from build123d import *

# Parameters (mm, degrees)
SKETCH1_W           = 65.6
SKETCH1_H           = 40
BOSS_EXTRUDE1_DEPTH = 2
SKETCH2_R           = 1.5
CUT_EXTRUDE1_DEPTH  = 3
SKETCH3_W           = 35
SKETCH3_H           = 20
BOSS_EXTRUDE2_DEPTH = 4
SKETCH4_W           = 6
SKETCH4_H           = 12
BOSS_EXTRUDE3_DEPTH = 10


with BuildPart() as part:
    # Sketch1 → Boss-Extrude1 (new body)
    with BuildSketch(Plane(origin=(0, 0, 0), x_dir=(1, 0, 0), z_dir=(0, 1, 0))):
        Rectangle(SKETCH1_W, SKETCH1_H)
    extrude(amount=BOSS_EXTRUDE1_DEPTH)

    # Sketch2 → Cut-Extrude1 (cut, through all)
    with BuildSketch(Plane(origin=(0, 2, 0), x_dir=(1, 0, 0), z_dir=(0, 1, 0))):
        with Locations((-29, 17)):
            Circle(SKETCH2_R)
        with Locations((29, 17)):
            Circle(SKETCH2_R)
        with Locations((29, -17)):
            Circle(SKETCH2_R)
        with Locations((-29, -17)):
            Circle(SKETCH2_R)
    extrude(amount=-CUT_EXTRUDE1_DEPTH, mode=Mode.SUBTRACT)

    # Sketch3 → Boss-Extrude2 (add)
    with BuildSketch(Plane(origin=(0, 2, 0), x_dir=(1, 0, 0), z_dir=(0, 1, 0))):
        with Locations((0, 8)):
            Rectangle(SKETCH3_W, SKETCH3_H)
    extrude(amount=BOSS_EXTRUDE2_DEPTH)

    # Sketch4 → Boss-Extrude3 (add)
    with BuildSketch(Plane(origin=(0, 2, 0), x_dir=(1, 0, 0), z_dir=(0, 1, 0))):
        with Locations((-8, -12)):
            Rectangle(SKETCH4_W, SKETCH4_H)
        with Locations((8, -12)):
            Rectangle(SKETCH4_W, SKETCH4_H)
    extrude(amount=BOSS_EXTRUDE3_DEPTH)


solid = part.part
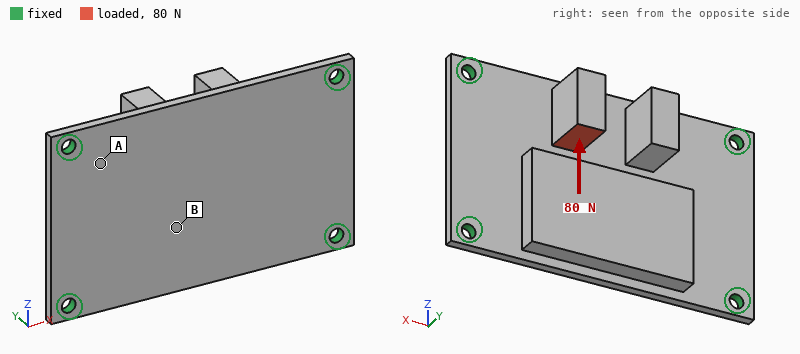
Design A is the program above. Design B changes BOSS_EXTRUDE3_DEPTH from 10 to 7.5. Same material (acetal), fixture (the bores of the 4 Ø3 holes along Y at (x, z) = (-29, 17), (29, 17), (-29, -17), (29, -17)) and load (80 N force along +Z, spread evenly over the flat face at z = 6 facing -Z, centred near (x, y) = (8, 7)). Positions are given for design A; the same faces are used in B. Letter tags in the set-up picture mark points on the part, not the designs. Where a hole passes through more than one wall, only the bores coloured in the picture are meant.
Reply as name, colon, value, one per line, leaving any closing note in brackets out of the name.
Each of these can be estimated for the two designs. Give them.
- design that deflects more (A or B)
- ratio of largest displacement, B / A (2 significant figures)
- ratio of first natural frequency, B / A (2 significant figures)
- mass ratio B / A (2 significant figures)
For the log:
design that deflects more: A
ratio of largest displacement, B / A: 0.71
ratio of first natural frequency, B / A: 1.1
mass ratio B / A: 0.96
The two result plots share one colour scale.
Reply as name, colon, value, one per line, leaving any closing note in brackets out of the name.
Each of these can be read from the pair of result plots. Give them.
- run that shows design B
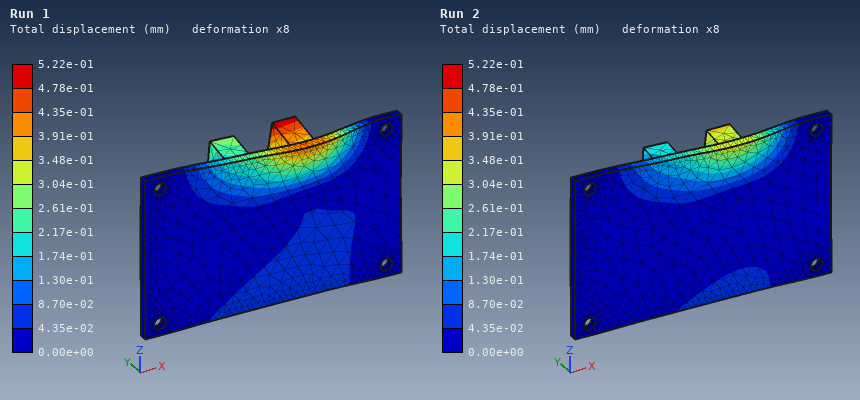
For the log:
run that shows design B: Run 2
